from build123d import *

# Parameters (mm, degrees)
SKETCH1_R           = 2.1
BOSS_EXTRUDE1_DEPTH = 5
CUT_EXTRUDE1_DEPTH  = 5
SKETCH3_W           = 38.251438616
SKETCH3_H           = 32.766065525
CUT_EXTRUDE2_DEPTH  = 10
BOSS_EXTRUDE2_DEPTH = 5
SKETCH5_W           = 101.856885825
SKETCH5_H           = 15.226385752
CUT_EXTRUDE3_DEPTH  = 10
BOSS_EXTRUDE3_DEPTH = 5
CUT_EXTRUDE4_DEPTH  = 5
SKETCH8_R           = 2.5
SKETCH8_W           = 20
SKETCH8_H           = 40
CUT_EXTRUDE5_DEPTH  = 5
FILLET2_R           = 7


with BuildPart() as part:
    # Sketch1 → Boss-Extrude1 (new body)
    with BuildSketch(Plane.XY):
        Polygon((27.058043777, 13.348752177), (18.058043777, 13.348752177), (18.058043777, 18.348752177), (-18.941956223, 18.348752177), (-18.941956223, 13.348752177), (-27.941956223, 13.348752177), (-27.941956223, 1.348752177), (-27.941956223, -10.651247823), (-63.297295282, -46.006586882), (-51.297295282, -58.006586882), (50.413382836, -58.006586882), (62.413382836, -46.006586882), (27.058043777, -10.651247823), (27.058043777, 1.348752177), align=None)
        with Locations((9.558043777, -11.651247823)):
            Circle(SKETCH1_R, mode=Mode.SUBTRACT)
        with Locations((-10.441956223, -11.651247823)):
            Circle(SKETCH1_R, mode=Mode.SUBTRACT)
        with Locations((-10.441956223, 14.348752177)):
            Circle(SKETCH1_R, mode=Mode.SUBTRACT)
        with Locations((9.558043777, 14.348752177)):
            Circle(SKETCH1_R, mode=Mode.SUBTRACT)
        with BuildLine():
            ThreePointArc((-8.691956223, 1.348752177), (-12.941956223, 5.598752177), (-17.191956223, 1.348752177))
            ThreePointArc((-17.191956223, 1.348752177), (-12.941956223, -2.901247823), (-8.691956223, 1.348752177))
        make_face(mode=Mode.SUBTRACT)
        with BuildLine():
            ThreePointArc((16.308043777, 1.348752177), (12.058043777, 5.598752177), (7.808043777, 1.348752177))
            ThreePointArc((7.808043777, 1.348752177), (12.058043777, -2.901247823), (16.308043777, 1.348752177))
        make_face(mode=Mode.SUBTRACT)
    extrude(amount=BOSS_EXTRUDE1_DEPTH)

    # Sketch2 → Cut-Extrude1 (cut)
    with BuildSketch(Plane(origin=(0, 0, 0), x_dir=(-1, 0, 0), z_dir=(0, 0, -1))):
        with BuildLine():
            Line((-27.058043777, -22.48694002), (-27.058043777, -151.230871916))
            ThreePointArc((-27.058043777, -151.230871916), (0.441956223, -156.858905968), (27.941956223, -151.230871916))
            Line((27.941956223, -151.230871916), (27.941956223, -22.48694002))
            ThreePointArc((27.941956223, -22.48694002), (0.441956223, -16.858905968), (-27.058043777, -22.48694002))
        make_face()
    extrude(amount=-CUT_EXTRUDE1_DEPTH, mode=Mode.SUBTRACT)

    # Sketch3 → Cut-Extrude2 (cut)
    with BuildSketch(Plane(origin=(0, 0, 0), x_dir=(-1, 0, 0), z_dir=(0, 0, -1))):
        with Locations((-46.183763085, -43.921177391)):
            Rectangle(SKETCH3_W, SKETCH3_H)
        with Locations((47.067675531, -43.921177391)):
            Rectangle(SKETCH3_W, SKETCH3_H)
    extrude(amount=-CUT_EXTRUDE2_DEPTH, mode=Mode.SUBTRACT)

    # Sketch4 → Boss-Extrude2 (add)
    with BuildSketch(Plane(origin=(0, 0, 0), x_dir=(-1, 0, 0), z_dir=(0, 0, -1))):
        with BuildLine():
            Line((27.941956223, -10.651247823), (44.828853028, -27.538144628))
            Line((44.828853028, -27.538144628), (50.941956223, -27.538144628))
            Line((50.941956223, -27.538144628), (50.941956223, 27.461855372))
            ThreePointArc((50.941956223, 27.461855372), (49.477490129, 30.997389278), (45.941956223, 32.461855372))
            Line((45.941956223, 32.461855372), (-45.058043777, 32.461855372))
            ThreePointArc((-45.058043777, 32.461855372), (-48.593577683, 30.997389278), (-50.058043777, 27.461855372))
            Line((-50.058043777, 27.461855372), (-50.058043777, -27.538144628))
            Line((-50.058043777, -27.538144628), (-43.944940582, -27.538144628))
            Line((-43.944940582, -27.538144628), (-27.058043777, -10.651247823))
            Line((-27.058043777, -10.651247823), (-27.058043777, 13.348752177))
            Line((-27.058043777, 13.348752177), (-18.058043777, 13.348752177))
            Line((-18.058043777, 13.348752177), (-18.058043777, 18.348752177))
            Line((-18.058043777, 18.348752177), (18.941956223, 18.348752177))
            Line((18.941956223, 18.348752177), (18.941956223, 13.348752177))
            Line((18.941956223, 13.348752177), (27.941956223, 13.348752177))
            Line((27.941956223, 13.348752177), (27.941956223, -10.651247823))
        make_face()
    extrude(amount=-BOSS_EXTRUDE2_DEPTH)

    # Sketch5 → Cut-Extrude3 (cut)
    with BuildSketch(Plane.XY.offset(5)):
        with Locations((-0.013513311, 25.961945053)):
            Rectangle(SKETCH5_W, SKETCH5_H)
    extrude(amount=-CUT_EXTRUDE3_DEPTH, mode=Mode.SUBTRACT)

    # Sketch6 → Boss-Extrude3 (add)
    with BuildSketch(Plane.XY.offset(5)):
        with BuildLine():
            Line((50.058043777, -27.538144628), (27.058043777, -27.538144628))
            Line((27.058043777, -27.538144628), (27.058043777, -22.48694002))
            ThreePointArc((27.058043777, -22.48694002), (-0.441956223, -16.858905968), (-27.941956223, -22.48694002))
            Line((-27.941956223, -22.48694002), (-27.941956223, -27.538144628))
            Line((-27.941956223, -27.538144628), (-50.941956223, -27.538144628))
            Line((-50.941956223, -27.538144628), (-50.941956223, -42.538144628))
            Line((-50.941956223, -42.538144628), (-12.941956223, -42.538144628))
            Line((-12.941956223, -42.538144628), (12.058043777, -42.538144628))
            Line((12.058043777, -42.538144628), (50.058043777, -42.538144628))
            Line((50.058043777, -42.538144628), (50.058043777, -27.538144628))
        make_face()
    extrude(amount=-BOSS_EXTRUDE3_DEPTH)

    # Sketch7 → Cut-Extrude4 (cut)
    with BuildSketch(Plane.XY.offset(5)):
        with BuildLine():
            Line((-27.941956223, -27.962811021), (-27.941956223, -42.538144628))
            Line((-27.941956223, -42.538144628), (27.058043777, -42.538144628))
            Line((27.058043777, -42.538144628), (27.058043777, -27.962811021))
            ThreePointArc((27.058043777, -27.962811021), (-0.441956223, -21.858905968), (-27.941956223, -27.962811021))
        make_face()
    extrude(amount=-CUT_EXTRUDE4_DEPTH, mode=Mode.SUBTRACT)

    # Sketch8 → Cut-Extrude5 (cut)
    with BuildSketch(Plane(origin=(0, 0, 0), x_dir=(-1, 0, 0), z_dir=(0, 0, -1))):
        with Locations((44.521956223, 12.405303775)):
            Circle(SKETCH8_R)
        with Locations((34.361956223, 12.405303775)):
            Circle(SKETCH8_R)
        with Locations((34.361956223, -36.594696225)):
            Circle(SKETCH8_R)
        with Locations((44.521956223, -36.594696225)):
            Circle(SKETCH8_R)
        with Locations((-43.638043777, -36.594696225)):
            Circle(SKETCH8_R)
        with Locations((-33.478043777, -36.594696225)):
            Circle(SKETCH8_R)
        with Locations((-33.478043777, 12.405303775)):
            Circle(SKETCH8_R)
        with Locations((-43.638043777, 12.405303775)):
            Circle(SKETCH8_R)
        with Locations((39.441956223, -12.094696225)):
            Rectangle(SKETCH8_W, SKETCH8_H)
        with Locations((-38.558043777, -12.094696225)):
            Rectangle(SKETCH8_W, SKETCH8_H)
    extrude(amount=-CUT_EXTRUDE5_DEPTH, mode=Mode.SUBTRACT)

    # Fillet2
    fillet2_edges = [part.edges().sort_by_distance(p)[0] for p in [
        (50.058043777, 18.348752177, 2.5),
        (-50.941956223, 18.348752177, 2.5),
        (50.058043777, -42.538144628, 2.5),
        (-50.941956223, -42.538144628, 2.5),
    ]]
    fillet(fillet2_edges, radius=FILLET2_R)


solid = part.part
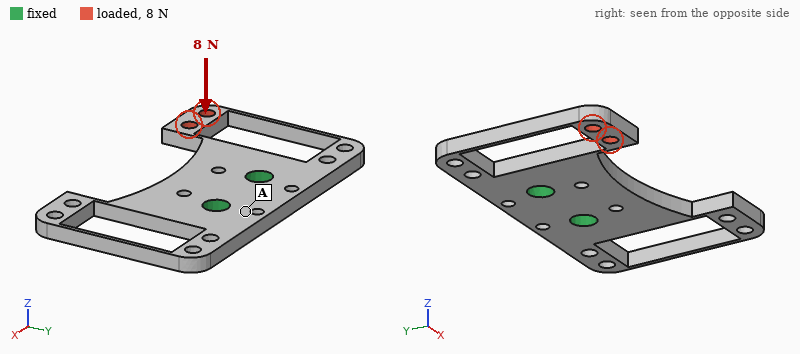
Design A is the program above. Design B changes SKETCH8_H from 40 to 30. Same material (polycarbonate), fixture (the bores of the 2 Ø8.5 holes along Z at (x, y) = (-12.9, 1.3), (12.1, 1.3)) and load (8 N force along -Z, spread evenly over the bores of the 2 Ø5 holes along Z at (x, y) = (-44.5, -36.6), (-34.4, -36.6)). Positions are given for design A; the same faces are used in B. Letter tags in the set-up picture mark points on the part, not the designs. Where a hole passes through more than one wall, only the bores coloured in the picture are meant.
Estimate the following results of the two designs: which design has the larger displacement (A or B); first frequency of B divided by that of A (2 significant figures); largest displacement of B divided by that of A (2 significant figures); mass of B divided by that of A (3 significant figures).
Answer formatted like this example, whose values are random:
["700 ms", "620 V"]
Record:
["A", "1.2", "0.52", "1.13"]
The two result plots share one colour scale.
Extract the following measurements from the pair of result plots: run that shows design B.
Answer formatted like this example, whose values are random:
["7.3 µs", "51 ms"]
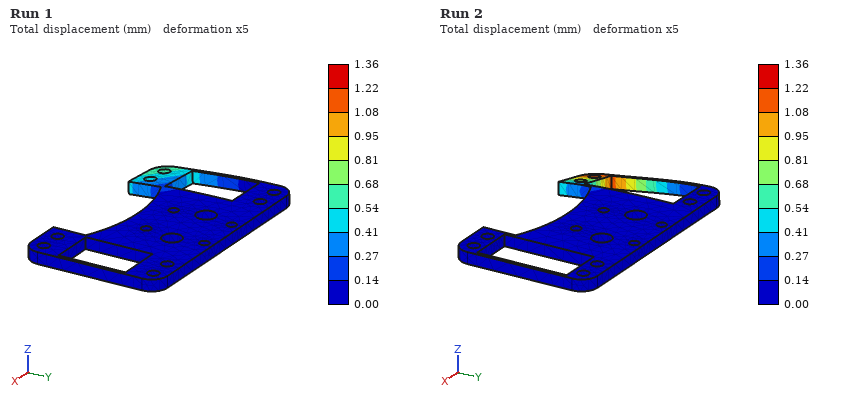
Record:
["Run 1"]
